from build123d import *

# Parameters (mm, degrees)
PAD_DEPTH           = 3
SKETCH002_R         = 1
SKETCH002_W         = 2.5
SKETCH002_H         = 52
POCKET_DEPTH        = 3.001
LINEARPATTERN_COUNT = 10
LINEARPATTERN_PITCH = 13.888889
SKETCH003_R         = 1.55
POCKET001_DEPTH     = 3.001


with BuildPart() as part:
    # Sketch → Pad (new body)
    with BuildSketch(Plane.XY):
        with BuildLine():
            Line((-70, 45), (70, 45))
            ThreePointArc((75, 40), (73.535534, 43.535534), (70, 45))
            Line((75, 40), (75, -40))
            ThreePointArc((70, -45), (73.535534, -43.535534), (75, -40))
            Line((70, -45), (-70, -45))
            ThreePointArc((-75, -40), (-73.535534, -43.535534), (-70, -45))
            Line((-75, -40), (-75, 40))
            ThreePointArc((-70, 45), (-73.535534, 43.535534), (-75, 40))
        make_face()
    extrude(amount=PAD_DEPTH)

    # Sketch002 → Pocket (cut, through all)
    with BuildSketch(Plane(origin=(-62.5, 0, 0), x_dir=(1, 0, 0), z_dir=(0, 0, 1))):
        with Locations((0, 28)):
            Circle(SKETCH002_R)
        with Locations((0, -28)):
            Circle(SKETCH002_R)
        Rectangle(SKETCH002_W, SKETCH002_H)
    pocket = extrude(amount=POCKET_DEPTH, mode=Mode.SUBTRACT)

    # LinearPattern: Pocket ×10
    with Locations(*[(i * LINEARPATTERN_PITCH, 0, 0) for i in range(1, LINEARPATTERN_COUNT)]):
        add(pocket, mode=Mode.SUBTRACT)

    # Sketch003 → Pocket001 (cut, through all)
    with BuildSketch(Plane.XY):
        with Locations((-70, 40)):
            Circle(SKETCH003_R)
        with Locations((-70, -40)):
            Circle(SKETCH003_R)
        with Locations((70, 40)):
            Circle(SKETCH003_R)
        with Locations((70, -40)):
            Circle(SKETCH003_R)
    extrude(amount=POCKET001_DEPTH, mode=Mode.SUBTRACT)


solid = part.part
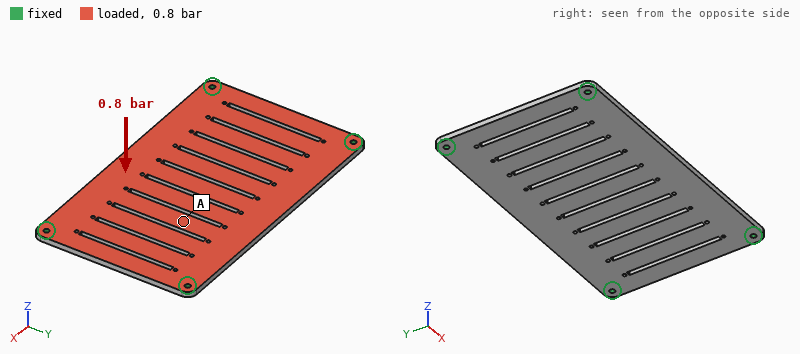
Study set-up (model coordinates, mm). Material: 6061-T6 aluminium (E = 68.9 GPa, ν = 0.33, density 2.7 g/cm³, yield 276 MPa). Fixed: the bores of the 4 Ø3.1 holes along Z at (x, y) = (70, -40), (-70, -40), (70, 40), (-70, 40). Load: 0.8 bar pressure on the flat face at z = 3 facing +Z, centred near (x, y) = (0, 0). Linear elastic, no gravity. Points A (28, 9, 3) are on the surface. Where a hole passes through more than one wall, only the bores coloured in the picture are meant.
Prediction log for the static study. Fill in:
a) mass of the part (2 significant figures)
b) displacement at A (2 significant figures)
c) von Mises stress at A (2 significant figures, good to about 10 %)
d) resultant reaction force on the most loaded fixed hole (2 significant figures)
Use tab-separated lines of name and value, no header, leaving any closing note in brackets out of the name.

mass of the part	98 g
displacement at A	0.94 mm
von Mises stress at A	27 MPa
resultant reaction force on the most loaded fixed hole	240 N
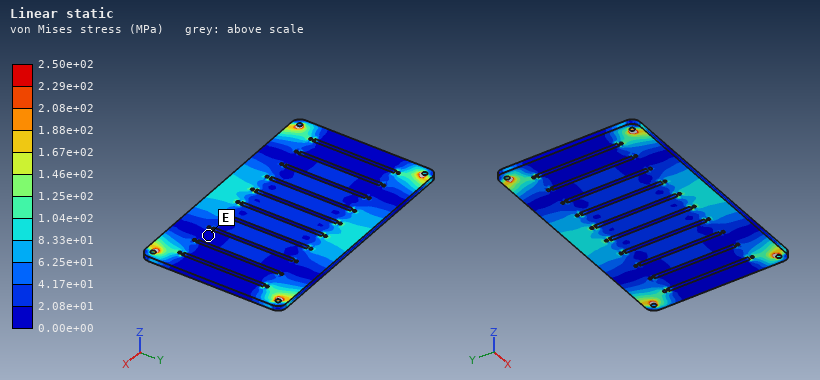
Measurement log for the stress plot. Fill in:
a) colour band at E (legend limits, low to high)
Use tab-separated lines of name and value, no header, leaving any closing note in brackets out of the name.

colour band at E	0.00e+00 to 2.08e+01 MPa
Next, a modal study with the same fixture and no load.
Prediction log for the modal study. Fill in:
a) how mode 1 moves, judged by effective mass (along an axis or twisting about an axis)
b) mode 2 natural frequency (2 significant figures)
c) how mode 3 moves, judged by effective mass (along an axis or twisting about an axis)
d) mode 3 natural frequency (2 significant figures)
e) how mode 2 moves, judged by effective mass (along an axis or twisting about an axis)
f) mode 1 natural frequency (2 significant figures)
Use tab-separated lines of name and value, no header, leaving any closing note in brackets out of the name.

how mode 1 moves, judged by effective mass	along Z
mode 2 natural frequency	1000 Hz
how mode 3 moves, judged by effective mass	twisting about Y
mode 3 natural frequency	1300 Hz
how mode 2 moves, judged by effective mass	twisting about X
mode 1 natural frequency	520 Hz
